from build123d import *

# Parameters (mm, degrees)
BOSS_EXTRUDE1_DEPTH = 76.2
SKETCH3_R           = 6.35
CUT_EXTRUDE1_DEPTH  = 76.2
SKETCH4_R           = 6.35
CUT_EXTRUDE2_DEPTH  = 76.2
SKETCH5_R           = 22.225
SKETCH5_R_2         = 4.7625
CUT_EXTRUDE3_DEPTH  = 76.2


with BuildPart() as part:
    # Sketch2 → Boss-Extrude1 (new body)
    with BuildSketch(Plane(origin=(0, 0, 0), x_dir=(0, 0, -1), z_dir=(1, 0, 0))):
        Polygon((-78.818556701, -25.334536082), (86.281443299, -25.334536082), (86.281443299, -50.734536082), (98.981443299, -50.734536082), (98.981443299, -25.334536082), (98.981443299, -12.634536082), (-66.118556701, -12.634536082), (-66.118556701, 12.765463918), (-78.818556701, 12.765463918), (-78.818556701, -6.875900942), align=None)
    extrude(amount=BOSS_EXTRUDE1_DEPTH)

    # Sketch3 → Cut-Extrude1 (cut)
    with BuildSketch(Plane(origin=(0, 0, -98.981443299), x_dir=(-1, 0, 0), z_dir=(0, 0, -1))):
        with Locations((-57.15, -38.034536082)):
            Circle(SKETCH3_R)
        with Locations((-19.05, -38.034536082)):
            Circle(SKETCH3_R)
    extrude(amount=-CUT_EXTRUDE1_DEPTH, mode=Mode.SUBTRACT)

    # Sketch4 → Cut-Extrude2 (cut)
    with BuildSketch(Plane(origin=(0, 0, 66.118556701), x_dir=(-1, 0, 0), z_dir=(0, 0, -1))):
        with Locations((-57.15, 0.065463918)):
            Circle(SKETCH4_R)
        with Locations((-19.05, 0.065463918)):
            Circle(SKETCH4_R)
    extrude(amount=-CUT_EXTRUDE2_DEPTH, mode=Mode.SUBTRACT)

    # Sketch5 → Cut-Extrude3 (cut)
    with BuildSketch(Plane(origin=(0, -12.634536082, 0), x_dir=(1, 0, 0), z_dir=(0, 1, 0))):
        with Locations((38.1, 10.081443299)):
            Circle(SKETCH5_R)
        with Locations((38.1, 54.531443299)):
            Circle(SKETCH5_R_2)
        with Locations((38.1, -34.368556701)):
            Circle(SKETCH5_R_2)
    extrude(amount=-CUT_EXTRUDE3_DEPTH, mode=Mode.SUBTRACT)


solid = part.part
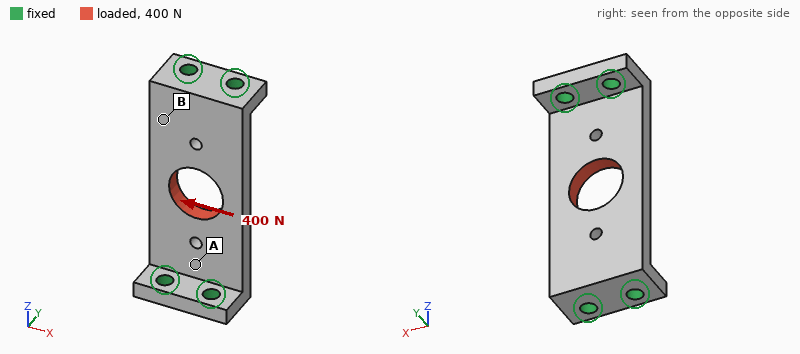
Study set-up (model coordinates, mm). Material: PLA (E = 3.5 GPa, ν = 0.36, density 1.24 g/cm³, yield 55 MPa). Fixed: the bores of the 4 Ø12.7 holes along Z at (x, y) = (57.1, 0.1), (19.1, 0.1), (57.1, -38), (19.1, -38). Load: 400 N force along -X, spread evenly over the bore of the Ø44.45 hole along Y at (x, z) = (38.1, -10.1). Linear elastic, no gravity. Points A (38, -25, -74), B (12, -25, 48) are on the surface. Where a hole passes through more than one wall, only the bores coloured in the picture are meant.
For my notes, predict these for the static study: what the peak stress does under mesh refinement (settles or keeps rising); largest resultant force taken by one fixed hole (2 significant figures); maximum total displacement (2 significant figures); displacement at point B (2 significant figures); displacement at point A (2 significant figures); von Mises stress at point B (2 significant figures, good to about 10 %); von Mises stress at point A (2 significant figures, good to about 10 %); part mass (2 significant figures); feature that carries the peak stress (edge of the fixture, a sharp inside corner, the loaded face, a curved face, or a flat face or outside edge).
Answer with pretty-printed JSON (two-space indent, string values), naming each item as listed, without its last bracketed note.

{
  "what the peak stress does under mesh refinement": "keeps rising",
  "largest resultant force taken by one fixed hole": "140 N",
  "maximum total displacement": "33 µm",
  "displacement at point B": "14 µm",
  "displacement at point A": "11 µm",
  "von Mises stress at point B": "0.26 MPa",
  "von Mises stress at point A": "0.71 MPa",
  "part mass": "240 g",
  "feature that carries the peak stress": "edge of the fixture"
}
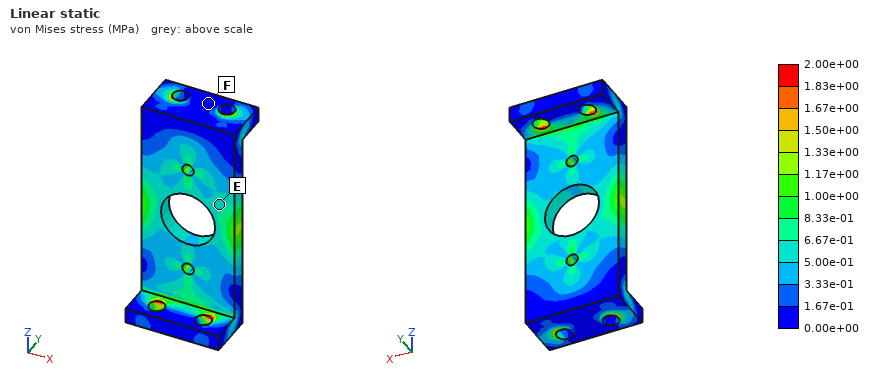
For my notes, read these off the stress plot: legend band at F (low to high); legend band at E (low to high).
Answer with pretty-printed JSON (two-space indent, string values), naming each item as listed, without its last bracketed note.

{
  "legend band at F": "0.00e+00 to 1.67e-01 MPa",
  "legend band at E": "5.00e-01 to 6.67e-01 MPa"
}
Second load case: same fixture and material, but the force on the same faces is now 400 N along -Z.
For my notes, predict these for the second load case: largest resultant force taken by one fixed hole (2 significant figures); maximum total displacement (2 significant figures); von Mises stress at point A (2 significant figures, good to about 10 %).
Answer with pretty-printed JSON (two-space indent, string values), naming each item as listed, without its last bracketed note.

{
  "largest resultant force taken by one fixed hole": "100 N",
  "maximum total displacement": "32 µm",
  "von Mises stress at point A": "0.26 MPa"
}
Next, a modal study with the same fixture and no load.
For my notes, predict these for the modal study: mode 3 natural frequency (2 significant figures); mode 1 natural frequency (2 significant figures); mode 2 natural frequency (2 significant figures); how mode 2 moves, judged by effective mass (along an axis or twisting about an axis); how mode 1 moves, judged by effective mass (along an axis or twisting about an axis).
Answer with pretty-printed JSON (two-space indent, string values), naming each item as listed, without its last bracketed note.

{
  "mode 3 natural frequency": "1800 Hz",
  "mode 1 natural frequency": "670 Hz",
  "mode 2 natural frequency": "1200 Hz",
  "how mode 2 moves, judged by effective mass": "twisting about Z",
  "how mode 1 moves, judged by effective mass": "along Y"
}
